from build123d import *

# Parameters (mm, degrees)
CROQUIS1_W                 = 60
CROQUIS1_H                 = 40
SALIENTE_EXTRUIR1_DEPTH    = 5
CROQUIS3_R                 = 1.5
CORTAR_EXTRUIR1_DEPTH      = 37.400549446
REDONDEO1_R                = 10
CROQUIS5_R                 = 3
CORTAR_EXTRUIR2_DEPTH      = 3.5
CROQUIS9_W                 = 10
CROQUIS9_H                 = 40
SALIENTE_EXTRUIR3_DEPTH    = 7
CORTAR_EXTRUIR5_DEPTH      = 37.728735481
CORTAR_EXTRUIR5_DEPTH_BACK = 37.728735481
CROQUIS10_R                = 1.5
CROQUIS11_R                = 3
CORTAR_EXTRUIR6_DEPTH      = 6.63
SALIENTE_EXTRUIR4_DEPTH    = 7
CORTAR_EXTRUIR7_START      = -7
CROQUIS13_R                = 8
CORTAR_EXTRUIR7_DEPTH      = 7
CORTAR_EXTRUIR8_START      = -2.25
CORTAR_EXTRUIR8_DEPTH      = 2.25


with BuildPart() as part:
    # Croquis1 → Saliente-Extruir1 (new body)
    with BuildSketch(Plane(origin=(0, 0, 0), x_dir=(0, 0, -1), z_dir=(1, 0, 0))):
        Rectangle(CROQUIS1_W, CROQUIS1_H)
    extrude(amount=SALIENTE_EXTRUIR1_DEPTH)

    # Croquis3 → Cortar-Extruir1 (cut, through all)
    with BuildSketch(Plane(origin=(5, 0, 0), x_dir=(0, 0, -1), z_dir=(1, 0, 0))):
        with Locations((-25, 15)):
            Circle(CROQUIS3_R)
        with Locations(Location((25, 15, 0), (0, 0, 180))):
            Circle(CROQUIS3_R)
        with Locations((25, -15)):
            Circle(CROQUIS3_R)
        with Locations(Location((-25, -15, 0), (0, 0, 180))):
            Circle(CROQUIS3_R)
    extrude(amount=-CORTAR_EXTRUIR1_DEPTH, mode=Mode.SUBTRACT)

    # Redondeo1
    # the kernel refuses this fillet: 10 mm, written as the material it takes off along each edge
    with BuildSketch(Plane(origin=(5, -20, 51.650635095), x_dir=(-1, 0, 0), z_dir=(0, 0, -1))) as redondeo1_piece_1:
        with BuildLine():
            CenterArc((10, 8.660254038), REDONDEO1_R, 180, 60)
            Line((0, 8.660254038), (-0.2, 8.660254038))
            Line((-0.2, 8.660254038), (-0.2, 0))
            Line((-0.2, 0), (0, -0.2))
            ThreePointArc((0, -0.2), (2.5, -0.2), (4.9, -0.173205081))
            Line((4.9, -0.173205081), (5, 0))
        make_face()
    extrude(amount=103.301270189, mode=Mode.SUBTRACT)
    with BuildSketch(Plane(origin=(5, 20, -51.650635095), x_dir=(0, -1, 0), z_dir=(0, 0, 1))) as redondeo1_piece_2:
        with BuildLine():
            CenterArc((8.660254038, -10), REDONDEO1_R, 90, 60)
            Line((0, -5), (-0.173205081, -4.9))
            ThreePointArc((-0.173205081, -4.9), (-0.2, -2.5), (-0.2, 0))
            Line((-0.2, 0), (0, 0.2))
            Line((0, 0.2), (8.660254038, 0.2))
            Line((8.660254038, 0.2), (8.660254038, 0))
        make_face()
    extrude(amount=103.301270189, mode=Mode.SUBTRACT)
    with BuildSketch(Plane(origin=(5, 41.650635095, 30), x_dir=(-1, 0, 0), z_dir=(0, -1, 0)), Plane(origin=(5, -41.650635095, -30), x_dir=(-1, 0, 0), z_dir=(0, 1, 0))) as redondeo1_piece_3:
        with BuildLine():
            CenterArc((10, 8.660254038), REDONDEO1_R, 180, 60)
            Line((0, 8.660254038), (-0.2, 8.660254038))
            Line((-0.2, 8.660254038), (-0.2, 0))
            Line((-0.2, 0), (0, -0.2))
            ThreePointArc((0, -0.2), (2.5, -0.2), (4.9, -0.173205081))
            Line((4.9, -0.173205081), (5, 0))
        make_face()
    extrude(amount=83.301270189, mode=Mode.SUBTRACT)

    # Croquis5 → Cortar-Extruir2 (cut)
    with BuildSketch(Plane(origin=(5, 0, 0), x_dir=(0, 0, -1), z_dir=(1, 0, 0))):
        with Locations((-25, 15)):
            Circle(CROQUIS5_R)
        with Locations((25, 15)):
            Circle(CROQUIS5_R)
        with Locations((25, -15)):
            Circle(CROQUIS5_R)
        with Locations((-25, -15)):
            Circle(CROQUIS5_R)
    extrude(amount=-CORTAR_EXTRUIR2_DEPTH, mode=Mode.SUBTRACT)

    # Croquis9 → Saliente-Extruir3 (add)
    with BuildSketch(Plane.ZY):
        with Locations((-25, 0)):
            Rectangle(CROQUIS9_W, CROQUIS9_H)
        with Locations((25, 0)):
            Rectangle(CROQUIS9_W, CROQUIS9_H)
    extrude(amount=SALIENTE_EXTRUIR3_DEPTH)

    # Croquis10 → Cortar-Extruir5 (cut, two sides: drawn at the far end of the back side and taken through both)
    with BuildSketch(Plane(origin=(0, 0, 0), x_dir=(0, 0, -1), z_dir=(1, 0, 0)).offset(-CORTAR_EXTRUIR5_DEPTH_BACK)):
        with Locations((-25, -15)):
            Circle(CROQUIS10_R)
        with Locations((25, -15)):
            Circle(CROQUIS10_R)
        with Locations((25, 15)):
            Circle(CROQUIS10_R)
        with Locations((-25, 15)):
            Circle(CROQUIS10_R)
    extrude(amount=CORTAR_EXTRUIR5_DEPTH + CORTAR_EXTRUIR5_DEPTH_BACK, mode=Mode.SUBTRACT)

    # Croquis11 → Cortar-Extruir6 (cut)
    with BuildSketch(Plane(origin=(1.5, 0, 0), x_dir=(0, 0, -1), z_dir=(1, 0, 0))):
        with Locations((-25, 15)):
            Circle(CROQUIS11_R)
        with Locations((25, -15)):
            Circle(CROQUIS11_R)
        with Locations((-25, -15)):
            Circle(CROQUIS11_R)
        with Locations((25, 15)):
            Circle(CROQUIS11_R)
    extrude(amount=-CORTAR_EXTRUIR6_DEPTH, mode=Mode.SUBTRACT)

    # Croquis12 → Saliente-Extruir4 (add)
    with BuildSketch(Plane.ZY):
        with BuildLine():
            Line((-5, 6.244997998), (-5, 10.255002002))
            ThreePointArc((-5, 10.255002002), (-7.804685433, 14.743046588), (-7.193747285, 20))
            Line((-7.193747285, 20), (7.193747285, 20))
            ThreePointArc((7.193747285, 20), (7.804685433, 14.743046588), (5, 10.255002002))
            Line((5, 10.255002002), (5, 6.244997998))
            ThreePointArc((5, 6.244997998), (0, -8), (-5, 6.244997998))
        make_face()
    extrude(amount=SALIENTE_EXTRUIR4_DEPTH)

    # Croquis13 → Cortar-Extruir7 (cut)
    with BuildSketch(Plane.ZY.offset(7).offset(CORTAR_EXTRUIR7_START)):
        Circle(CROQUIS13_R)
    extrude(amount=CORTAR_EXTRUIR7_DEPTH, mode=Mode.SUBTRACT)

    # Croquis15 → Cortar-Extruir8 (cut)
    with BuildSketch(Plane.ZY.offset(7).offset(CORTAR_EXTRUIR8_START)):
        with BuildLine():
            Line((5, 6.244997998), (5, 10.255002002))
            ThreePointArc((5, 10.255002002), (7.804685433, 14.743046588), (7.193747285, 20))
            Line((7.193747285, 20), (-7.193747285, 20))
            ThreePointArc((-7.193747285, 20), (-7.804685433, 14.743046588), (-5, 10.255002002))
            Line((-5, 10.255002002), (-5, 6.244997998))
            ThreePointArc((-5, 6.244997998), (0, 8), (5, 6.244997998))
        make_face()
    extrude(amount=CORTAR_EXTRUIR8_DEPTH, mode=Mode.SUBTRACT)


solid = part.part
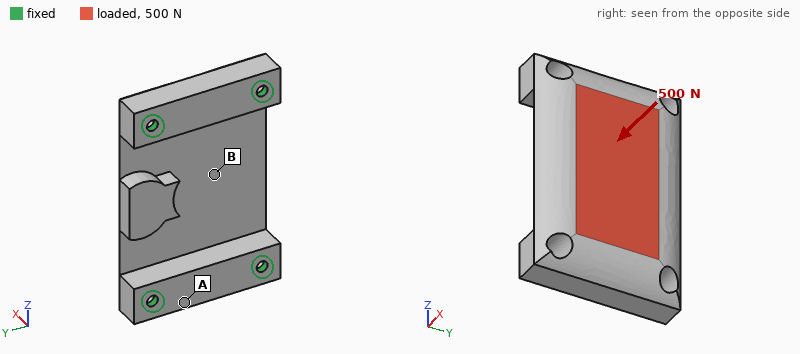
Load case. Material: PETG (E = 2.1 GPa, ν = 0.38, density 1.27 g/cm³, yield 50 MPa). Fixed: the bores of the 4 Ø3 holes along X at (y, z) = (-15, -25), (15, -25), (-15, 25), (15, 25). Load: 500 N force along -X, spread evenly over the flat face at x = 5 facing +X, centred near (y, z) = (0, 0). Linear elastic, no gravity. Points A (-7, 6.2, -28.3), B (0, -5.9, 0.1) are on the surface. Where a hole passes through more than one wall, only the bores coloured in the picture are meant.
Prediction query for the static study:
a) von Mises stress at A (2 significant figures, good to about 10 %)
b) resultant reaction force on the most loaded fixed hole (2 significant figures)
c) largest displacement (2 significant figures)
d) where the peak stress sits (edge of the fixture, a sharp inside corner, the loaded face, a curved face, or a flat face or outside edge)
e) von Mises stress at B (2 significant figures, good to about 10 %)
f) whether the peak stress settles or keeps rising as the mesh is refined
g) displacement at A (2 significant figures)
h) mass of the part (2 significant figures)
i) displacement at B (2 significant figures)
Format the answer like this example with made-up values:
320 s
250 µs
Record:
2.5 MPa
190 N
0.27 mm
edge of the fixture
6.0 MPa
keeps rising
0.044 mm
19 g
0.27 mm
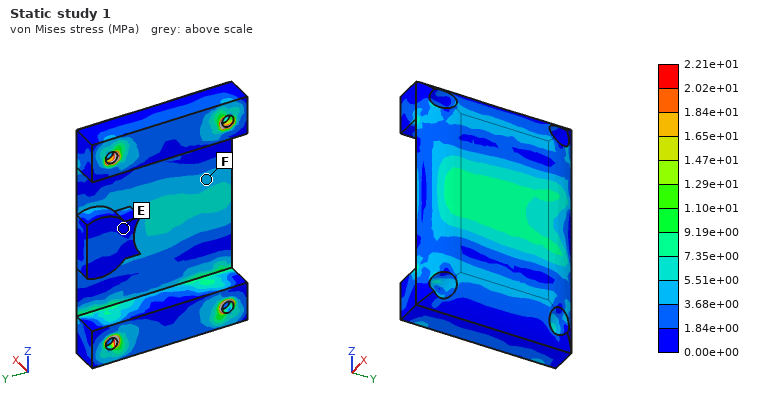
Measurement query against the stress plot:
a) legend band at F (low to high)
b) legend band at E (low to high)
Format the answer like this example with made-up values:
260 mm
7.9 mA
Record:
3.68e+00 to 5.51e+00 MPa
0.00e+00 to 1.84e+00 MPa
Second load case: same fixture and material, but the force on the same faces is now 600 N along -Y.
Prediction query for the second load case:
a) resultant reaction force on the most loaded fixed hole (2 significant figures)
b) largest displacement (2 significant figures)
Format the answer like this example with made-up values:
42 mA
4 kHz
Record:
190 N
0.11 mm
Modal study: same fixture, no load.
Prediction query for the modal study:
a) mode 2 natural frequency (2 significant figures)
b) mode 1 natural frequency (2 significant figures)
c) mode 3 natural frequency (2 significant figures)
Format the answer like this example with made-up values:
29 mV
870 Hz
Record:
2300 Hz
2300 Hz
2900 Hz
